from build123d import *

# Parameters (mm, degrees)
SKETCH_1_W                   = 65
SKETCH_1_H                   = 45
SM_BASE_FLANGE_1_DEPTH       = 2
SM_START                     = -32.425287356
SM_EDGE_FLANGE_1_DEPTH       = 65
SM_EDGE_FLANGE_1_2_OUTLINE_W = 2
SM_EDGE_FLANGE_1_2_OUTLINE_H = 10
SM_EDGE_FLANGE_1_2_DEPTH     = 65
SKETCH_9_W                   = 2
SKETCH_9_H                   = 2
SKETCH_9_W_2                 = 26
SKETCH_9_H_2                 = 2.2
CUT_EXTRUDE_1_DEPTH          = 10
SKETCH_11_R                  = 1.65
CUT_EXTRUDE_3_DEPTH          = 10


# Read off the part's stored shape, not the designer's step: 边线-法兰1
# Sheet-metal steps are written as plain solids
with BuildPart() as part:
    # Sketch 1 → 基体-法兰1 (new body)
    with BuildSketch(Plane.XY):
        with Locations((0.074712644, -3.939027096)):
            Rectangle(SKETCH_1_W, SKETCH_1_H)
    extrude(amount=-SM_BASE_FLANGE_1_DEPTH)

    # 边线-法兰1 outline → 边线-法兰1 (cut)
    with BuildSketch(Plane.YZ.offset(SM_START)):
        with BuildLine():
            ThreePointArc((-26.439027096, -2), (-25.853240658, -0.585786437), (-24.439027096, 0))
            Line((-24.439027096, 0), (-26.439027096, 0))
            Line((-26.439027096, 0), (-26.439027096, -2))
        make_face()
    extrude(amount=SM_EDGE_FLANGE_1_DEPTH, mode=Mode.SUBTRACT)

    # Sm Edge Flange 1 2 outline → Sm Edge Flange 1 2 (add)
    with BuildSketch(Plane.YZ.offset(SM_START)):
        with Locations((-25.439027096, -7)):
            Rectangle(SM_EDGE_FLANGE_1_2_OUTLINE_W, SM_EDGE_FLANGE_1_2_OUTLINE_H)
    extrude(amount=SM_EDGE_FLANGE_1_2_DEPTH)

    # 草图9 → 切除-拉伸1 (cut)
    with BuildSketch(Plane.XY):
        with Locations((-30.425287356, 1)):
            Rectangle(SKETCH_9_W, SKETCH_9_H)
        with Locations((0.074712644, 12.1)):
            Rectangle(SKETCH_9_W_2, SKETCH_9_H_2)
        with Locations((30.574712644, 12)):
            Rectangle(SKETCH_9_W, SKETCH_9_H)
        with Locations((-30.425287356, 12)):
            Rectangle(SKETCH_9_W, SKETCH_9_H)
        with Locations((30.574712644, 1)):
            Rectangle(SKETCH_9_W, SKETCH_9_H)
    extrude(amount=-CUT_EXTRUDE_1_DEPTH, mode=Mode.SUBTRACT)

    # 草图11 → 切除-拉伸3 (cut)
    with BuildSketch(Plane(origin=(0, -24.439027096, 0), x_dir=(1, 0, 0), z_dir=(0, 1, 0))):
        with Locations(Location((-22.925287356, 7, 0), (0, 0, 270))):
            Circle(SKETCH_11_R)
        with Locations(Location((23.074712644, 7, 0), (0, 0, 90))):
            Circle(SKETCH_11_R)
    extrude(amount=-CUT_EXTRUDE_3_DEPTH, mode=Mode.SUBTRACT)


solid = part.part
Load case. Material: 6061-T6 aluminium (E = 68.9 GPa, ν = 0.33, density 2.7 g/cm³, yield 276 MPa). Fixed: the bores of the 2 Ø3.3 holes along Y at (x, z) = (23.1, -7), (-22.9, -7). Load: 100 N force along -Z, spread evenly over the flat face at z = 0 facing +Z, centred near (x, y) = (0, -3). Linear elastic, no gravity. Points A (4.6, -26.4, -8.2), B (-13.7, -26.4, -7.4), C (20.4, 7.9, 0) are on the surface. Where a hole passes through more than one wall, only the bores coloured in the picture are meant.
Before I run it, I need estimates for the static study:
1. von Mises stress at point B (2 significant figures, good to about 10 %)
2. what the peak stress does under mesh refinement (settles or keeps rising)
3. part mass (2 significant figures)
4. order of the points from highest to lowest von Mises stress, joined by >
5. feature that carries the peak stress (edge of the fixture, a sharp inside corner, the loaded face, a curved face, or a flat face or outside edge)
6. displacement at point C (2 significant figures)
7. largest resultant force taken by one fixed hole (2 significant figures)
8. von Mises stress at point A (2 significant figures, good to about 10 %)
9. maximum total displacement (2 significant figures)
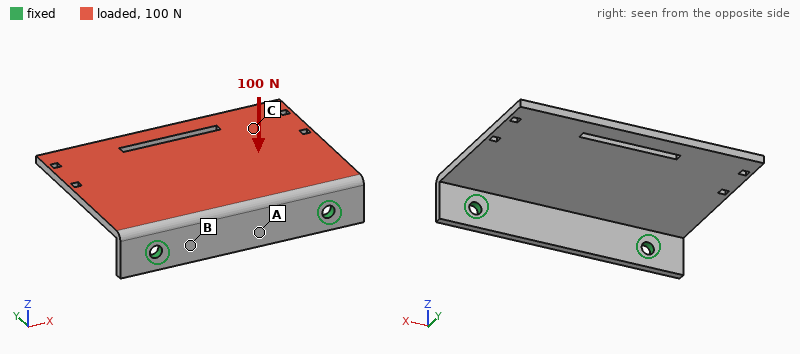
37 MPa
keeps rising
19 g
B > A > C
edge of the fixture
0.45 mm
53 N
19 MPa
0.64 mm
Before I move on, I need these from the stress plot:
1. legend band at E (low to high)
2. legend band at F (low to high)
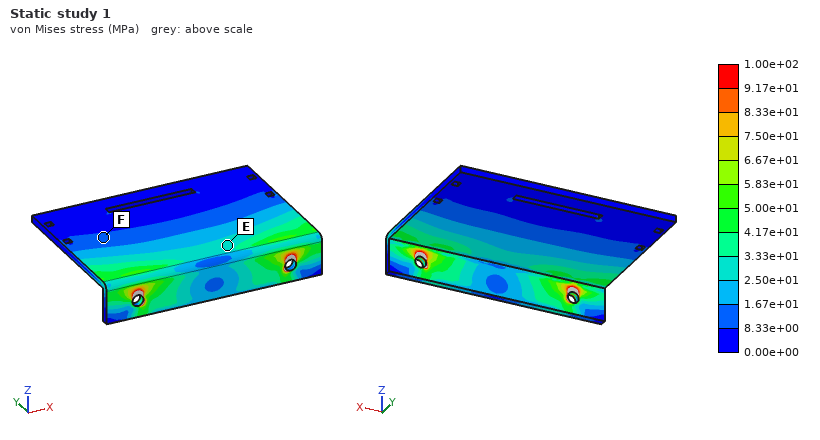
2.50e+01 to 3.33e+01 MPa
8.33e+00 to 1.67e+01 MPa
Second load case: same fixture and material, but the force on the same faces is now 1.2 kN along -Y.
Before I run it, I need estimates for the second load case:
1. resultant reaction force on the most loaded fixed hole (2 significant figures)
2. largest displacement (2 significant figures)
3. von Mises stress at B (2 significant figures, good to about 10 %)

600 N
0.89 mm
60 MPa
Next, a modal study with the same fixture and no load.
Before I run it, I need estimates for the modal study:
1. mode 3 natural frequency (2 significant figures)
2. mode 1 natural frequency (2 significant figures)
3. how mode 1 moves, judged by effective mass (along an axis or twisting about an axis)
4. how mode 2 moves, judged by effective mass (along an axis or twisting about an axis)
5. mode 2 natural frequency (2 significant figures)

3500 Hz
650 Hz
along Z
twisting about Y
1400 Hz
